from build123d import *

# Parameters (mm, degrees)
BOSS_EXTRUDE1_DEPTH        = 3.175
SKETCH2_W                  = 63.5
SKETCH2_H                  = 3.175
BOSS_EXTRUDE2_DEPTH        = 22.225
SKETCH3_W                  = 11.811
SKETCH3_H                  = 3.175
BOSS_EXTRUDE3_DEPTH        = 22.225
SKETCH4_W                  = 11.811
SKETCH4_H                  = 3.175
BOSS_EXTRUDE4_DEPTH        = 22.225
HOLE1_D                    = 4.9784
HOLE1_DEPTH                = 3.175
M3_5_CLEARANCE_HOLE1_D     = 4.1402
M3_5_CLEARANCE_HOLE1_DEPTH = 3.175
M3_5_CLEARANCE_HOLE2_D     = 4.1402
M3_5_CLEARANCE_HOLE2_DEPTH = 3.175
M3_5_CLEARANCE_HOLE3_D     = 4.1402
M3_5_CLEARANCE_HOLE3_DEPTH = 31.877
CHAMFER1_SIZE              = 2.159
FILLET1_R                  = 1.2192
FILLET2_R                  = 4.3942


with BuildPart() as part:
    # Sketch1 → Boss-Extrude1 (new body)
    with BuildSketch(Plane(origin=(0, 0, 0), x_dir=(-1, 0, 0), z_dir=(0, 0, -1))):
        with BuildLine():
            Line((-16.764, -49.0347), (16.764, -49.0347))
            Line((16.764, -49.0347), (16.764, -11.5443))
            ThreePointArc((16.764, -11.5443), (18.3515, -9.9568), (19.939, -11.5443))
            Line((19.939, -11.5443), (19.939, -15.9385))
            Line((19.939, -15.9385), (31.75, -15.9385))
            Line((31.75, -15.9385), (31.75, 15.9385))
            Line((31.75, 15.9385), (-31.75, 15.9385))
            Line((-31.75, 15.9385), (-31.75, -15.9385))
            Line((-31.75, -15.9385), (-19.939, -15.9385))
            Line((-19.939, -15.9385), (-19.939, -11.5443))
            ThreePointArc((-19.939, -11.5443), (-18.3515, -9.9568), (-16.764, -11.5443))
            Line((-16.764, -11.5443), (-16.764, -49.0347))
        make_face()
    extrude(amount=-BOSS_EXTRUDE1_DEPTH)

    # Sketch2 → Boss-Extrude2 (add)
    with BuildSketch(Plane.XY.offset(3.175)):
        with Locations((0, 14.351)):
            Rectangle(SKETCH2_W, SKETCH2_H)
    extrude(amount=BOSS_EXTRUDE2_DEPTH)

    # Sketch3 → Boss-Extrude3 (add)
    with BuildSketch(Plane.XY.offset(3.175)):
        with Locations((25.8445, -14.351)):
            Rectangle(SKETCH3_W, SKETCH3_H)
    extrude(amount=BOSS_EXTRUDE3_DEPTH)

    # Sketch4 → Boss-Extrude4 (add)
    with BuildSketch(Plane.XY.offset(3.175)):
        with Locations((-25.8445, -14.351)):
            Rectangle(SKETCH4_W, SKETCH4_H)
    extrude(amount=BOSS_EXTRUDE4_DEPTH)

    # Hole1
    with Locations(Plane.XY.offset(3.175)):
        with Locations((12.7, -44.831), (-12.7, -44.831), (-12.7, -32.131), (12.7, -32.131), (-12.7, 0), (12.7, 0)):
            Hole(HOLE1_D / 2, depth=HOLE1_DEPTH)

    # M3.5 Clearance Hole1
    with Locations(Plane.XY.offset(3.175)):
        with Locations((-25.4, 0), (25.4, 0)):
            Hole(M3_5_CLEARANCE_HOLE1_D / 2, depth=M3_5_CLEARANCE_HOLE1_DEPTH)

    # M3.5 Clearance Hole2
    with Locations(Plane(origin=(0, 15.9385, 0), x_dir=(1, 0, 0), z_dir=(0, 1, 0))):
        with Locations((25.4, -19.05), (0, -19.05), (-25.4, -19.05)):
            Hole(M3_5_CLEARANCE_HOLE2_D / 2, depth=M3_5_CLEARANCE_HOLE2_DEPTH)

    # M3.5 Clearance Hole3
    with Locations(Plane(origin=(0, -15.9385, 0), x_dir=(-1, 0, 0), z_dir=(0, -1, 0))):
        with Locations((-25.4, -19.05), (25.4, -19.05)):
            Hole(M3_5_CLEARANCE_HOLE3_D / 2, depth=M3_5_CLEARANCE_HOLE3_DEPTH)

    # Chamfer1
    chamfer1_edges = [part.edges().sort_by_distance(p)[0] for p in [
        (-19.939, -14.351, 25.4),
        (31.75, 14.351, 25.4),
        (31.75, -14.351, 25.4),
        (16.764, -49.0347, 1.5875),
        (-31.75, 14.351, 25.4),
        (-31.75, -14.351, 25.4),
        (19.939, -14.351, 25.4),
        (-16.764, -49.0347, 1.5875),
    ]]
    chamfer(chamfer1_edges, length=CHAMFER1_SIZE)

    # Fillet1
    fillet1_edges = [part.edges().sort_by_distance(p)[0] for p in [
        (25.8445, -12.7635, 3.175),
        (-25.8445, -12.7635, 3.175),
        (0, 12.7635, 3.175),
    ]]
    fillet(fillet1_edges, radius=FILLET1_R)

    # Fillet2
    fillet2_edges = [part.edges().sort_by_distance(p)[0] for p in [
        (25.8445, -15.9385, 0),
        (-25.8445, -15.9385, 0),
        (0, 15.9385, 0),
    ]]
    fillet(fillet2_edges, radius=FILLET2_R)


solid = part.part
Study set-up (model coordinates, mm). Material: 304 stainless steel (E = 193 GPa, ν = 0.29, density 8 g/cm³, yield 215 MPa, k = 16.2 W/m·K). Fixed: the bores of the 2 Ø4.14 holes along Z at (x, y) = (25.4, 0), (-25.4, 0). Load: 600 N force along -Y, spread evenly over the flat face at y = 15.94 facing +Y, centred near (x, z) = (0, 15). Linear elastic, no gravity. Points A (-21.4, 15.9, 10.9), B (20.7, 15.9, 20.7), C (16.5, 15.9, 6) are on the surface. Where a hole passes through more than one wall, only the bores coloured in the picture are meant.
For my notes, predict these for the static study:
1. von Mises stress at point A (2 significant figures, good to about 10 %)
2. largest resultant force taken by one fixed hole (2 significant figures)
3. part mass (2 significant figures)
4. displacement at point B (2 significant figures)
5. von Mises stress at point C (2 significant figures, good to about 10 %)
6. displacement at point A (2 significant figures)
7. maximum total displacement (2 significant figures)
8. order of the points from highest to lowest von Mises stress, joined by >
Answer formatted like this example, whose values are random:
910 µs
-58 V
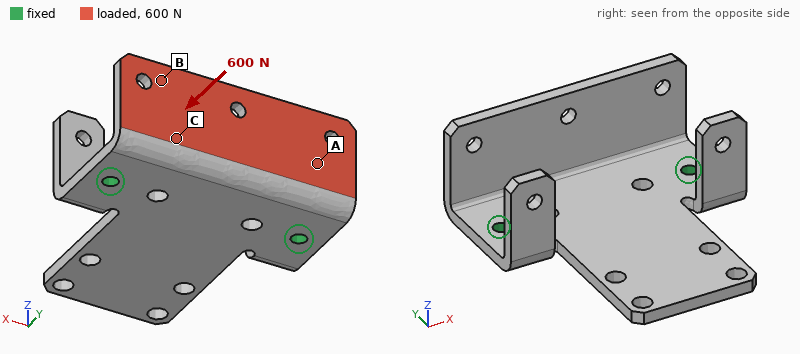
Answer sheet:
25 MPa
300 N
120 g
0.10 mm
44 MPa
0.058 mm
0.13 mm
C > A > B
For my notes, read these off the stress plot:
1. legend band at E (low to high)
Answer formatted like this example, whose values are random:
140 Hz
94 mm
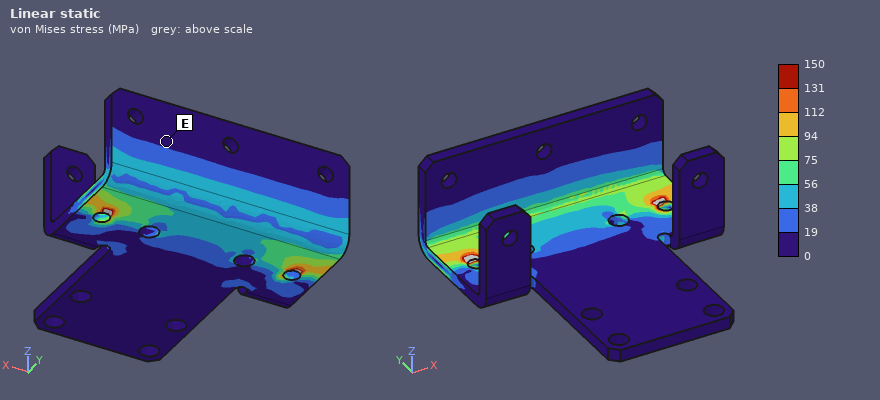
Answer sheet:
0 to 19 MPa
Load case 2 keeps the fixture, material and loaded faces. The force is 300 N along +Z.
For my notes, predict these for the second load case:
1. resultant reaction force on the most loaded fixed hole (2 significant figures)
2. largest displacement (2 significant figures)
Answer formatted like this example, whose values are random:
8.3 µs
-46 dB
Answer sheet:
150 N
42 µm
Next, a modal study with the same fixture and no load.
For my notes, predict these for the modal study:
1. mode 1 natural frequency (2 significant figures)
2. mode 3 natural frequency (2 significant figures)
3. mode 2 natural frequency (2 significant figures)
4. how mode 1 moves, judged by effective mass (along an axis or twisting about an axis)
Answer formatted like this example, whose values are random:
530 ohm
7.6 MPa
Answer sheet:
990 Hz
2700 Hz
2200 Hz
along Z
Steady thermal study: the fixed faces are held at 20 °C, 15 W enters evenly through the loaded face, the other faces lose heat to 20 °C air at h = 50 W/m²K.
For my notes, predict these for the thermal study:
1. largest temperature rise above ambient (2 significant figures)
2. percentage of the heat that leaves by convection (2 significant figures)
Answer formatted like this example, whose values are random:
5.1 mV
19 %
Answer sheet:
76 K
67 %
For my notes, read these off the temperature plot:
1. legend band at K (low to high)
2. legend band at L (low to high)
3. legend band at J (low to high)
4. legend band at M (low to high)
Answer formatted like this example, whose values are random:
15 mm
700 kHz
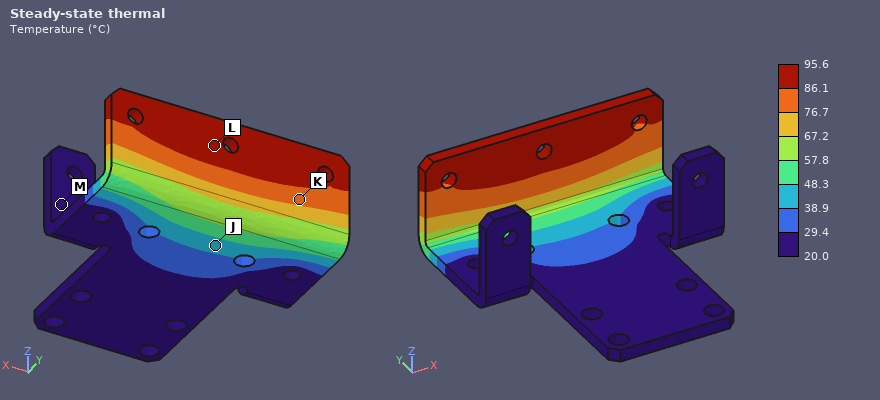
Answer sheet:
76.7 to 86.1 °C
86.1 to 95.6 °C
38.9 to 48.3 °C
20.0 to 29.4 °C
